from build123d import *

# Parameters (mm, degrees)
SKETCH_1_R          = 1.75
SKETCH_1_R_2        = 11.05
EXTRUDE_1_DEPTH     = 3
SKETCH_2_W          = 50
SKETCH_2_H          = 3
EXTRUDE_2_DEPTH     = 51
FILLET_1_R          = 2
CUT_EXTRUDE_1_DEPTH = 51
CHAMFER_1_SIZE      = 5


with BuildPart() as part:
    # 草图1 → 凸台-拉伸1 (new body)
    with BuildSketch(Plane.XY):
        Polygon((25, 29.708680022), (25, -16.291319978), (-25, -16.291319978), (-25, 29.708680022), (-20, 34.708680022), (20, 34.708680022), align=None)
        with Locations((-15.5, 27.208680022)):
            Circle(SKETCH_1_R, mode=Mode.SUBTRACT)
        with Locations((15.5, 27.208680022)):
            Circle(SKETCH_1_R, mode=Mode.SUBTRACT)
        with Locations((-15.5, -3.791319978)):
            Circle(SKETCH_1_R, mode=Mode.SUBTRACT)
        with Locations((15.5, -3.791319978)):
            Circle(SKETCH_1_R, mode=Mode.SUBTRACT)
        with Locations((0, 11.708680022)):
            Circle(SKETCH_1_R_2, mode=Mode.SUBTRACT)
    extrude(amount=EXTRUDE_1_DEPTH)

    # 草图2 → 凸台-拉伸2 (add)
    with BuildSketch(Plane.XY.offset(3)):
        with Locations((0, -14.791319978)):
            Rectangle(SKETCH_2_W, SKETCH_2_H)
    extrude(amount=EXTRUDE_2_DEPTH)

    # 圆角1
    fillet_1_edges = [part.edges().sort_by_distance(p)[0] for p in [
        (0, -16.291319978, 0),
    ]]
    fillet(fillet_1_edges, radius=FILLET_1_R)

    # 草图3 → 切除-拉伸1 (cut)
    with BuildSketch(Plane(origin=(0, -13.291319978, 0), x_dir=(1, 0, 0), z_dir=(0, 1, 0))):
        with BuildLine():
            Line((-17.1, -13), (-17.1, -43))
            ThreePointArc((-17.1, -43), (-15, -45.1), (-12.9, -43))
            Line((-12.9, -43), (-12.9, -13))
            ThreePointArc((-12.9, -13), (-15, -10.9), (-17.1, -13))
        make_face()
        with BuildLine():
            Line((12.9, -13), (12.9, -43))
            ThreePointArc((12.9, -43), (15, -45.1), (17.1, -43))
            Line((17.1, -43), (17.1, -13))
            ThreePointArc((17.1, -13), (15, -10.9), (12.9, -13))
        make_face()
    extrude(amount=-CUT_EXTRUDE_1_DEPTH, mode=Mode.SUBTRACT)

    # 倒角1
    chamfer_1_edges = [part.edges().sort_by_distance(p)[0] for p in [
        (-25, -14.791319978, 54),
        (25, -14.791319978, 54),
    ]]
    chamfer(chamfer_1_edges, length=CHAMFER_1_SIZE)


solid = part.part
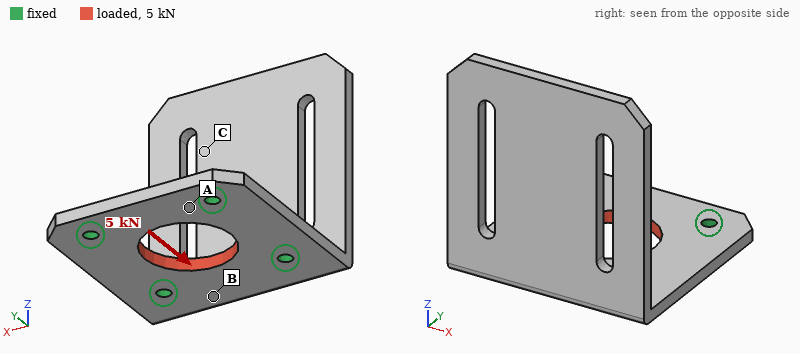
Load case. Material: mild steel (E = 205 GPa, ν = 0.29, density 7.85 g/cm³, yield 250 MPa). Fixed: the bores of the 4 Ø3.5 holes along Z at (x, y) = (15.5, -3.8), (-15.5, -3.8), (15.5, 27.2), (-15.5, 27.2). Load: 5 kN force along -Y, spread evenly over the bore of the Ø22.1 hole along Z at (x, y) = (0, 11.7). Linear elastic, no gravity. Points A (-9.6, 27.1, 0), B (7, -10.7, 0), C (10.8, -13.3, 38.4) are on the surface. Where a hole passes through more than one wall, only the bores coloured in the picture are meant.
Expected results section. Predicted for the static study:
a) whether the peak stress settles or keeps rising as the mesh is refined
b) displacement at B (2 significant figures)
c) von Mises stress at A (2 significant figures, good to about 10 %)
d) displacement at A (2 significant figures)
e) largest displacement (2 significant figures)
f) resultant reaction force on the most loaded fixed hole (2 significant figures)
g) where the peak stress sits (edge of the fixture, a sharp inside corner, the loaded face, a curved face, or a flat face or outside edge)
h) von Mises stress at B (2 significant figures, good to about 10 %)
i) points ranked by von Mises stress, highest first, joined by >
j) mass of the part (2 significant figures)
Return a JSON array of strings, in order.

["keeps rising", "1.7 µm", "30 MPa", "1.9 µm", "4.3 µm", "1.3 kN", "edge of the fixture", "18 MPa", "A > B > C", "100 g"]
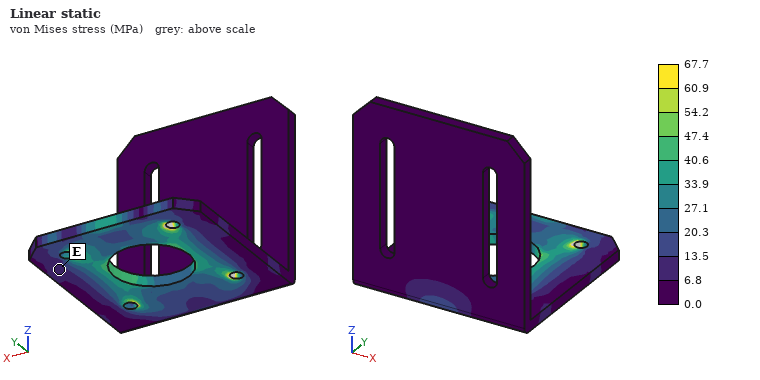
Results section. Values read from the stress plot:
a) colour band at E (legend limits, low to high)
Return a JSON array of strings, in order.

["6.8 to 13.5 MPa"]
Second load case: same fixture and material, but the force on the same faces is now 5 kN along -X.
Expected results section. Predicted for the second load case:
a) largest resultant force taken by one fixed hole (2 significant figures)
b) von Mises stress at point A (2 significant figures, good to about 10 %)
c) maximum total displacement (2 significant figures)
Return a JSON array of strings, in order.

["1.3 kN", "29 MPa", "3.8 µm"]
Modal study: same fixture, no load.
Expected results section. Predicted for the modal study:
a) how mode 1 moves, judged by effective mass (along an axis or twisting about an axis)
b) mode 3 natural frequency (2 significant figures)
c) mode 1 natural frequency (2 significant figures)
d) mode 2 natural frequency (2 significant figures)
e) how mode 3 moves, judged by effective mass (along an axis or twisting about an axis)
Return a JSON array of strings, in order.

["along Y", "2800 Hz", "690 Hz", "1900 Hz", "along X"]
